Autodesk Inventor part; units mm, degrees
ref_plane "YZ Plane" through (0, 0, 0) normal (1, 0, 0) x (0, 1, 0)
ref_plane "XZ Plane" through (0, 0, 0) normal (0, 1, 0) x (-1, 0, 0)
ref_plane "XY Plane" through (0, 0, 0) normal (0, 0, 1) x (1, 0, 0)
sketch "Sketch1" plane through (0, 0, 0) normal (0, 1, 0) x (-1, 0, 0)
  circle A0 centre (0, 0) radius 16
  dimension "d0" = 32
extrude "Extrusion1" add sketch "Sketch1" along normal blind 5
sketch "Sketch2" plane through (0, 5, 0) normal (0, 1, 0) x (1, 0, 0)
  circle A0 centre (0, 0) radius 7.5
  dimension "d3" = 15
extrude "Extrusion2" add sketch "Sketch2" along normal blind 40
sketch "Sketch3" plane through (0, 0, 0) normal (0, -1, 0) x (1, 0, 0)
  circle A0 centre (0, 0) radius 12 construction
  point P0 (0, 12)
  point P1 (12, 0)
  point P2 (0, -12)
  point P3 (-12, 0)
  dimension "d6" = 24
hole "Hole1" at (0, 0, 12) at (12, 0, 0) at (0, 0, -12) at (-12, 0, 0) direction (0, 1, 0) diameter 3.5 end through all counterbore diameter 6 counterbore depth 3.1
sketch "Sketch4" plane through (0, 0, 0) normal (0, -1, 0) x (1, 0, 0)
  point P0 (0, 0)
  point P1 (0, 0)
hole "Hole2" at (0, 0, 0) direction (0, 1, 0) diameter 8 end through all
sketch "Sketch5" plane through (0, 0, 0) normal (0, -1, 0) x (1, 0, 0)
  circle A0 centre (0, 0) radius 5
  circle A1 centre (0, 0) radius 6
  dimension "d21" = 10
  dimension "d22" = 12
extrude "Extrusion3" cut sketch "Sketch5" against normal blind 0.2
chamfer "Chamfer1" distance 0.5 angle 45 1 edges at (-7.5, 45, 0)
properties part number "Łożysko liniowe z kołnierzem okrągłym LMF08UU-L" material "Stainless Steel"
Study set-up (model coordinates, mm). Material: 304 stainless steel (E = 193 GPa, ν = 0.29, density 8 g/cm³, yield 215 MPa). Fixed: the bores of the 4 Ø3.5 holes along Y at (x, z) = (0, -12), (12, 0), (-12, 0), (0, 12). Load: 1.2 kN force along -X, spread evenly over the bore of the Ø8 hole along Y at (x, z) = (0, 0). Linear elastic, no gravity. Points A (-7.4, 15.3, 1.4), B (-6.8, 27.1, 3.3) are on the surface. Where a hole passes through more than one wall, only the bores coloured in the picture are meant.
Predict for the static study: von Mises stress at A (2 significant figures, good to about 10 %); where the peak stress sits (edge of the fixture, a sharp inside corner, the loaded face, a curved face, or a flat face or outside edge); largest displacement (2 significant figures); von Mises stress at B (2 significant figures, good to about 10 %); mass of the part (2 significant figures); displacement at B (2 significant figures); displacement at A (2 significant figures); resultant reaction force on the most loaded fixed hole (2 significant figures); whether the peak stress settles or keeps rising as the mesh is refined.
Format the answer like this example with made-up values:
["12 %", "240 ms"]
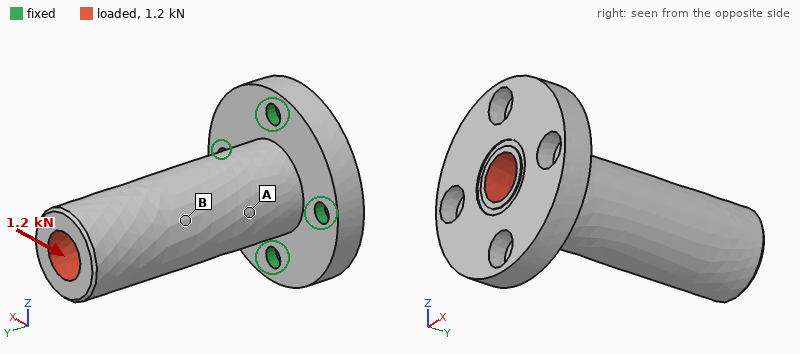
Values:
["36 MPa", "edge of the fixture", "44 µm", "13 MPa", "67 g", "24 µm", "12 µm", "980 N", "keeps rising"]
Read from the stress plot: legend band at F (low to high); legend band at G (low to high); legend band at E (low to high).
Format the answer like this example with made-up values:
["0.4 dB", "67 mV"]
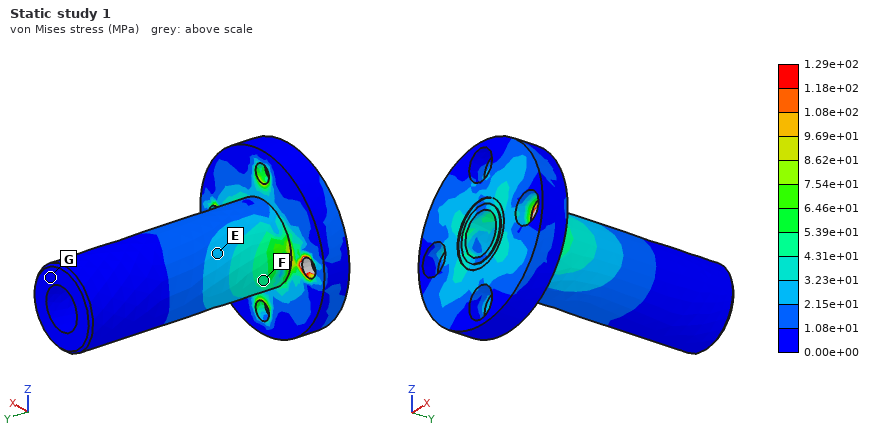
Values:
["4.31e+01 to 5.39e+01 MPa", "0.00e+00 to 1.08e+01 MPa", "2.15e+01 to 3.23e+01 MPa"]
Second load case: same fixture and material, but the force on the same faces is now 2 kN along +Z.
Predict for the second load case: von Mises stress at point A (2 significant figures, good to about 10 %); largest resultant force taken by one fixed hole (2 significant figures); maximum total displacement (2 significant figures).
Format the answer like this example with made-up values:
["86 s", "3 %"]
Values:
["29 MPa", "1.6 kN", "74 µm"]
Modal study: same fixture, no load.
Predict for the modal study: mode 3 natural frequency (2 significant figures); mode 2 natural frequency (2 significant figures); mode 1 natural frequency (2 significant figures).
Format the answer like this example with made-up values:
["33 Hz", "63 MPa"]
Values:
["18 kHz", "4700 Hz", "4700 Hz"]
